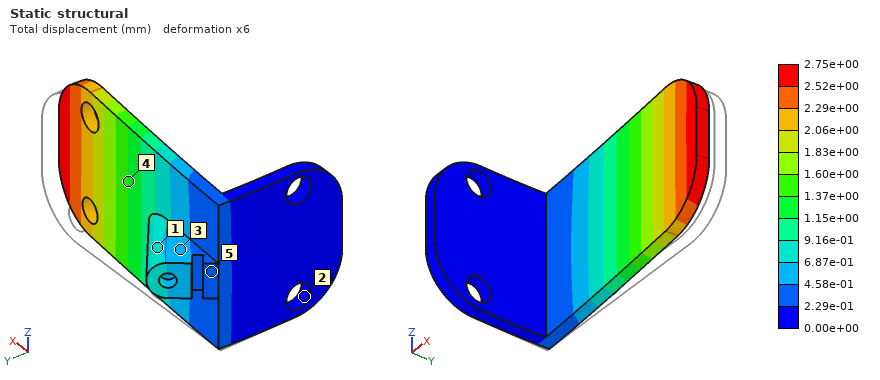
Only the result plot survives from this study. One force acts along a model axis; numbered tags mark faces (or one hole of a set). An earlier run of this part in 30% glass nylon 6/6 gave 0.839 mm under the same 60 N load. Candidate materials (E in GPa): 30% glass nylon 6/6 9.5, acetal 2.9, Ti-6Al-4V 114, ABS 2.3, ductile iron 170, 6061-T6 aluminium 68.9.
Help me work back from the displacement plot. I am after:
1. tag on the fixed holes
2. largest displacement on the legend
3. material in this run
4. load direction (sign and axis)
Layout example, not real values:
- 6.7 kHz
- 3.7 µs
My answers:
- 2
- 2.75e+00 mm
- acetal
- -Y
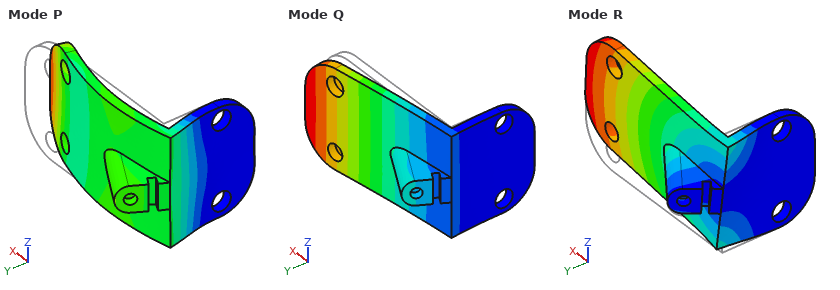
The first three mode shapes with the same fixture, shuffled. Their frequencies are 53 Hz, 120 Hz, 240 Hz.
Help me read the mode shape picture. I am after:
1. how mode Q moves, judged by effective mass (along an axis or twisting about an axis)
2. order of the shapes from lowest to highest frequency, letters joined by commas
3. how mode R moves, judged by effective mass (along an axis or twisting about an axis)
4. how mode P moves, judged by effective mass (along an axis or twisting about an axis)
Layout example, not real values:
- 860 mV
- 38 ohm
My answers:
- along Y
- Q, R, P
- along Z
- along X
